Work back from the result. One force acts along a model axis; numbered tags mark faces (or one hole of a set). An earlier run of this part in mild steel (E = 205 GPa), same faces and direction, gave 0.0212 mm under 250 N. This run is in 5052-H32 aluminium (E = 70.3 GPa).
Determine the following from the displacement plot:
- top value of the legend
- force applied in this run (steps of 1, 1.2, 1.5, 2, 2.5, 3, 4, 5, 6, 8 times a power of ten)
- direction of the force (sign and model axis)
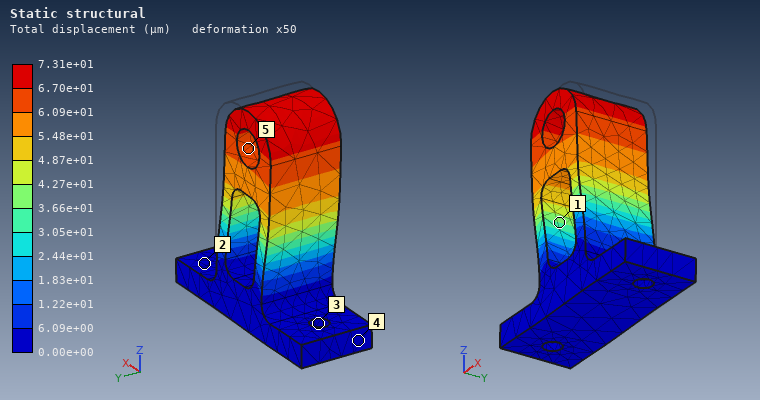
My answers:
7.31e+01 µm
300 N
-X
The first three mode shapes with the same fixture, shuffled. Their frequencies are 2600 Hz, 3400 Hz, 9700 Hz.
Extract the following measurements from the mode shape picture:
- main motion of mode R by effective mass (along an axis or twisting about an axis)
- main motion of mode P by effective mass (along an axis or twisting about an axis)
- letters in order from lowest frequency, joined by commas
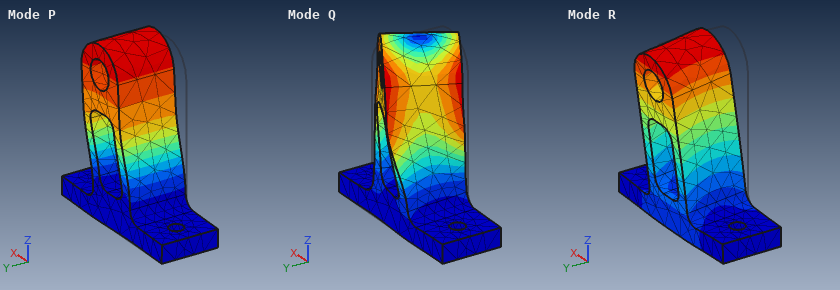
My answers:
along Y
along X
R, P, Q
